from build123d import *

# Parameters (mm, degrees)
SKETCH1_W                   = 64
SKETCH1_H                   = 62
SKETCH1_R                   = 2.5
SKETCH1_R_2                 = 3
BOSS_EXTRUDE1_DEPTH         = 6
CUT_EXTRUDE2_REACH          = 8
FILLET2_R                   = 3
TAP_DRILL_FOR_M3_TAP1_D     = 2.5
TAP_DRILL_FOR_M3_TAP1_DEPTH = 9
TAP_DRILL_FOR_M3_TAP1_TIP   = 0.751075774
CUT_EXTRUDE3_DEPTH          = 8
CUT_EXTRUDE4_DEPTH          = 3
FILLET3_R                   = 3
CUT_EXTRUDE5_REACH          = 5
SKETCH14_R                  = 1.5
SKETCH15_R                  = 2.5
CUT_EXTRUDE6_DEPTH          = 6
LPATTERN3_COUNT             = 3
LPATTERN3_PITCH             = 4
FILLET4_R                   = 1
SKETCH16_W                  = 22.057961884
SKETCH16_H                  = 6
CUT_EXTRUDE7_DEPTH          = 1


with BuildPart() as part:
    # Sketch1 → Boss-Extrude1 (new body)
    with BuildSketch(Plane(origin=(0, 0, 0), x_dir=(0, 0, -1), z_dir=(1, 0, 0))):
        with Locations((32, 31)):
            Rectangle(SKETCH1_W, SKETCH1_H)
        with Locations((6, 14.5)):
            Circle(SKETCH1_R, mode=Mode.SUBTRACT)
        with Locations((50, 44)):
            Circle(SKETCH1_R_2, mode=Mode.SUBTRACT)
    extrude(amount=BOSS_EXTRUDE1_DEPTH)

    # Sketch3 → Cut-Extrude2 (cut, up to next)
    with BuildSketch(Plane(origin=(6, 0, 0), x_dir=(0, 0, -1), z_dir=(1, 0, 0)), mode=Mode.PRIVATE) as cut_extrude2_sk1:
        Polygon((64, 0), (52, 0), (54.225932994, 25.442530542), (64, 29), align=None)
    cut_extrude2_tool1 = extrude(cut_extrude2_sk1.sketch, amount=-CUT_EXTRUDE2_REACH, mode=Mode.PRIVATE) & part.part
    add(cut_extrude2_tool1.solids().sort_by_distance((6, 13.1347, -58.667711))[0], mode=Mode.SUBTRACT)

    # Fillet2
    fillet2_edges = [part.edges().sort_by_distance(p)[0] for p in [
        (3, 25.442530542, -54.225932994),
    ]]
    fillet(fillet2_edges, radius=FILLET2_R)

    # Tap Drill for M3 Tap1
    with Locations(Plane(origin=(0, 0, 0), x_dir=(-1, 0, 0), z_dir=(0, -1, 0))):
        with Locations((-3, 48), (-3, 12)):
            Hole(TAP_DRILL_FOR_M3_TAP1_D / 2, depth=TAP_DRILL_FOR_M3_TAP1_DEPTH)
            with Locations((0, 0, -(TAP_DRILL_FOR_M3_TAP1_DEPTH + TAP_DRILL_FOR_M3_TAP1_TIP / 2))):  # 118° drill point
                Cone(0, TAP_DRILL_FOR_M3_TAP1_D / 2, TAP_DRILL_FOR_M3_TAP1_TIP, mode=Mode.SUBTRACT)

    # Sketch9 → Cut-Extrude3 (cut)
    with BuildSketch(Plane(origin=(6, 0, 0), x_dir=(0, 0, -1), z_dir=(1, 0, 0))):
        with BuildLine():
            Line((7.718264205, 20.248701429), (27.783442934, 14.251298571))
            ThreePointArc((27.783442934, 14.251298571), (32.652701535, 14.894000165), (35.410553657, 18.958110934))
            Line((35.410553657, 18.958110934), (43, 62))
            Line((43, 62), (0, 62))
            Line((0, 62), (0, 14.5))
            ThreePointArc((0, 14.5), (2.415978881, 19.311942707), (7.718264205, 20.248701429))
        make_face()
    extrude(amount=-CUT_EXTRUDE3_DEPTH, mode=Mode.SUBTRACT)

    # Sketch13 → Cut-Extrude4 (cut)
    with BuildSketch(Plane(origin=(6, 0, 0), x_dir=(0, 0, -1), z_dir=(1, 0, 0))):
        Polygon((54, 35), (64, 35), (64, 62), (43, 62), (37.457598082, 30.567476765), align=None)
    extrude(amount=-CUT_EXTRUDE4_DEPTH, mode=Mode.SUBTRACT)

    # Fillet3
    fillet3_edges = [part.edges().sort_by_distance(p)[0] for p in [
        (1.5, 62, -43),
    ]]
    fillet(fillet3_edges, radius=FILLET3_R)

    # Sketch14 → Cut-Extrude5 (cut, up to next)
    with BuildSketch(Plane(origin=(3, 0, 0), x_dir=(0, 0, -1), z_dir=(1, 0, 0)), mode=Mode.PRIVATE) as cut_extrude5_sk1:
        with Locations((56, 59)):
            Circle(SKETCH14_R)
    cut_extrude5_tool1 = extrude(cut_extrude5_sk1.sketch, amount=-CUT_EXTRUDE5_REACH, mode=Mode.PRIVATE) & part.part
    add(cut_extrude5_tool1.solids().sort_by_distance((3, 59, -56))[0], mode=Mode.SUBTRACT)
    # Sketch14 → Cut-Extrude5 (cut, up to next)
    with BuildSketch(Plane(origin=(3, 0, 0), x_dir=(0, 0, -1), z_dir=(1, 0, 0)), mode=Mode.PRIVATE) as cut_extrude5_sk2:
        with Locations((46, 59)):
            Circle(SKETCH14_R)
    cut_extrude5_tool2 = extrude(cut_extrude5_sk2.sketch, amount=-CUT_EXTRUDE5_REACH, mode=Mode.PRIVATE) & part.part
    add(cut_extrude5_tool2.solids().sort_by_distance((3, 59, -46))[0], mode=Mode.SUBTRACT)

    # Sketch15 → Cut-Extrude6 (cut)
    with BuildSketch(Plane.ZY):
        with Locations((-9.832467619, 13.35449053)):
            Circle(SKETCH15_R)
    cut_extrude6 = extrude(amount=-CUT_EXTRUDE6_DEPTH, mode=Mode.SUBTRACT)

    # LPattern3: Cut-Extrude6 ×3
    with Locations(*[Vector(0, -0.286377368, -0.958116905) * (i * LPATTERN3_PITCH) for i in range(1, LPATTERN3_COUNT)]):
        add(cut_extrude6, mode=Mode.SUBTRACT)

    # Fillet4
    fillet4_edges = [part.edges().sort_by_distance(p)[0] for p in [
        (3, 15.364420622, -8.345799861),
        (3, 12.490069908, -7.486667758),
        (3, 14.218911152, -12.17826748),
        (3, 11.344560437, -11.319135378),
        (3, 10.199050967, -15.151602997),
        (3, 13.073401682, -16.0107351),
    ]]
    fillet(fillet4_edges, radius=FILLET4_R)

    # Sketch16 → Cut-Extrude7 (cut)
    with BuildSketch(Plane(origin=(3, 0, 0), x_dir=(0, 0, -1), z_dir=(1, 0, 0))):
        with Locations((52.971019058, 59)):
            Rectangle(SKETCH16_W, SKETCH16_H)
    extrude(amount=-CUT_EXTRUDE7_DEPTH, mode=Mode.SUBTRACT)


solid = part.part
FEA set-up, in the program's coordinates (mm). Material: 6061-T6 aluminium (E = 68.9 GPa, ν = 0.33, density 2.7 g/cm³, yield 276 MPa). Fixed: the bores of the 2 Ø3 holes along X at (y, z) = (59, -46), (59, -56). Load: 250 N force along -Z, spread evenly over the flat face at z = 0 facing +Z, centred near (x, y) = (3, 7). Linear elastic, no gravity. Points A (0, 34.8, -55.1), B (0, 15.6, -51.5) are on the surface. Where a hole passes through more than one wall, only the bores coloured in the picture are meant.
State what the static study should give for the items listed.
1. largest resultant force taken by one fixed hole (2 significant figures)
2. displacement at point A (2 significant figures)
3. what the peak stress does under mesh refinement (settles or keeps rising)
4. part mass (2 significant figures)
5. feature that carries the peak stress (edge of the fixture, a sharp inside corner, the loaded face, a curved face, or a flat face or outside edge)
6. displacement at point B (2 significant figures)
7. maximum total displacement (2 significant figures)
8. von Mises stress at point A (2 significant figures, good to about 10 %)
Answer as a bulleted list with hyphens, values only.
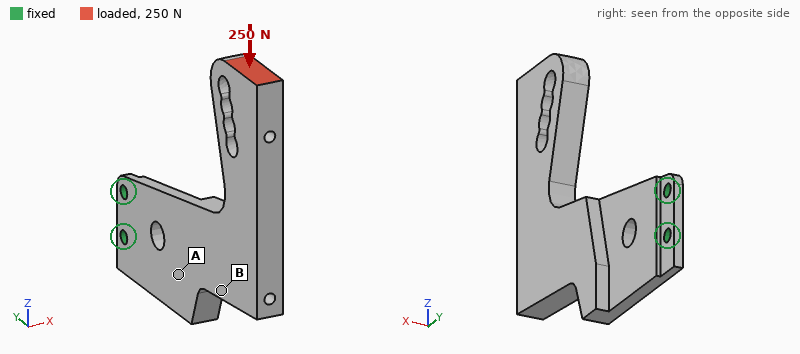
- 1.1 kN
- 0.039 mm
- keeps rising
- 24 g
- edge of the fixture
- 0.082 mm
- 0.17 mm
- 16 MPa
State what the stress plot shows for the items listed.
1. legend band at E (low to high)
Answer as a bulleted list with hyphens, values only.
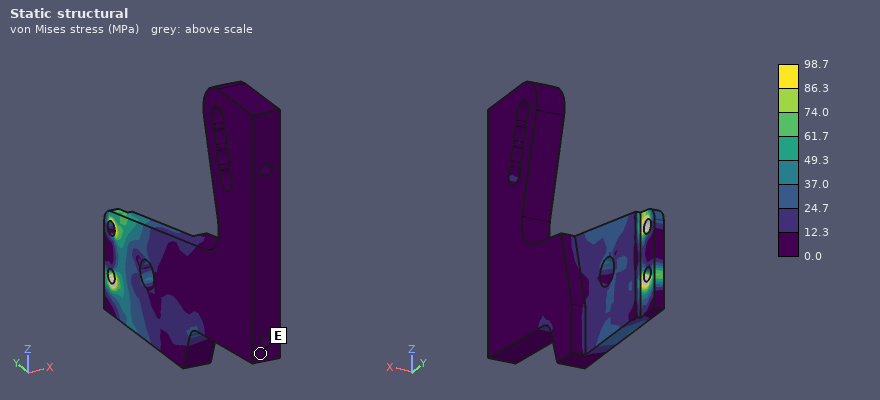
- 0.0 to 12.3 MPa
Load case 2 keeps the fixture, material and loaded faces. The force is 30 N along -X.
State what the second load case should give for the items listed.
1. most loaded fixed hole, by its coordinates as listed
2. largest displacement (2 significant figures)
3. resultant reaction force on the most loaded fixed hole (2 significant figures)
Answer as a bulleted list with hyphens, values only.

- (59, -46)
- 1.1 mm
- 120 N
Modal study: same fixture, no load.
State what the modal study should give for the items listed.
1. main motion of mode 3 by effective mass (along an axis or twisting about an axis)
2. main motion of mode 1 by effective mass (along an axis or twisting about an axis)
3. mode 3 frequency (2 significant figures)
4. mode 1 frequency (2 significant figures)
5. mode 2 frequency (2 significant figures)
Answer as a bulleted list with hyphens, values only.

- along Z
- along X
- 1700 Hz
- 290 Hz
- 1100 Hz
